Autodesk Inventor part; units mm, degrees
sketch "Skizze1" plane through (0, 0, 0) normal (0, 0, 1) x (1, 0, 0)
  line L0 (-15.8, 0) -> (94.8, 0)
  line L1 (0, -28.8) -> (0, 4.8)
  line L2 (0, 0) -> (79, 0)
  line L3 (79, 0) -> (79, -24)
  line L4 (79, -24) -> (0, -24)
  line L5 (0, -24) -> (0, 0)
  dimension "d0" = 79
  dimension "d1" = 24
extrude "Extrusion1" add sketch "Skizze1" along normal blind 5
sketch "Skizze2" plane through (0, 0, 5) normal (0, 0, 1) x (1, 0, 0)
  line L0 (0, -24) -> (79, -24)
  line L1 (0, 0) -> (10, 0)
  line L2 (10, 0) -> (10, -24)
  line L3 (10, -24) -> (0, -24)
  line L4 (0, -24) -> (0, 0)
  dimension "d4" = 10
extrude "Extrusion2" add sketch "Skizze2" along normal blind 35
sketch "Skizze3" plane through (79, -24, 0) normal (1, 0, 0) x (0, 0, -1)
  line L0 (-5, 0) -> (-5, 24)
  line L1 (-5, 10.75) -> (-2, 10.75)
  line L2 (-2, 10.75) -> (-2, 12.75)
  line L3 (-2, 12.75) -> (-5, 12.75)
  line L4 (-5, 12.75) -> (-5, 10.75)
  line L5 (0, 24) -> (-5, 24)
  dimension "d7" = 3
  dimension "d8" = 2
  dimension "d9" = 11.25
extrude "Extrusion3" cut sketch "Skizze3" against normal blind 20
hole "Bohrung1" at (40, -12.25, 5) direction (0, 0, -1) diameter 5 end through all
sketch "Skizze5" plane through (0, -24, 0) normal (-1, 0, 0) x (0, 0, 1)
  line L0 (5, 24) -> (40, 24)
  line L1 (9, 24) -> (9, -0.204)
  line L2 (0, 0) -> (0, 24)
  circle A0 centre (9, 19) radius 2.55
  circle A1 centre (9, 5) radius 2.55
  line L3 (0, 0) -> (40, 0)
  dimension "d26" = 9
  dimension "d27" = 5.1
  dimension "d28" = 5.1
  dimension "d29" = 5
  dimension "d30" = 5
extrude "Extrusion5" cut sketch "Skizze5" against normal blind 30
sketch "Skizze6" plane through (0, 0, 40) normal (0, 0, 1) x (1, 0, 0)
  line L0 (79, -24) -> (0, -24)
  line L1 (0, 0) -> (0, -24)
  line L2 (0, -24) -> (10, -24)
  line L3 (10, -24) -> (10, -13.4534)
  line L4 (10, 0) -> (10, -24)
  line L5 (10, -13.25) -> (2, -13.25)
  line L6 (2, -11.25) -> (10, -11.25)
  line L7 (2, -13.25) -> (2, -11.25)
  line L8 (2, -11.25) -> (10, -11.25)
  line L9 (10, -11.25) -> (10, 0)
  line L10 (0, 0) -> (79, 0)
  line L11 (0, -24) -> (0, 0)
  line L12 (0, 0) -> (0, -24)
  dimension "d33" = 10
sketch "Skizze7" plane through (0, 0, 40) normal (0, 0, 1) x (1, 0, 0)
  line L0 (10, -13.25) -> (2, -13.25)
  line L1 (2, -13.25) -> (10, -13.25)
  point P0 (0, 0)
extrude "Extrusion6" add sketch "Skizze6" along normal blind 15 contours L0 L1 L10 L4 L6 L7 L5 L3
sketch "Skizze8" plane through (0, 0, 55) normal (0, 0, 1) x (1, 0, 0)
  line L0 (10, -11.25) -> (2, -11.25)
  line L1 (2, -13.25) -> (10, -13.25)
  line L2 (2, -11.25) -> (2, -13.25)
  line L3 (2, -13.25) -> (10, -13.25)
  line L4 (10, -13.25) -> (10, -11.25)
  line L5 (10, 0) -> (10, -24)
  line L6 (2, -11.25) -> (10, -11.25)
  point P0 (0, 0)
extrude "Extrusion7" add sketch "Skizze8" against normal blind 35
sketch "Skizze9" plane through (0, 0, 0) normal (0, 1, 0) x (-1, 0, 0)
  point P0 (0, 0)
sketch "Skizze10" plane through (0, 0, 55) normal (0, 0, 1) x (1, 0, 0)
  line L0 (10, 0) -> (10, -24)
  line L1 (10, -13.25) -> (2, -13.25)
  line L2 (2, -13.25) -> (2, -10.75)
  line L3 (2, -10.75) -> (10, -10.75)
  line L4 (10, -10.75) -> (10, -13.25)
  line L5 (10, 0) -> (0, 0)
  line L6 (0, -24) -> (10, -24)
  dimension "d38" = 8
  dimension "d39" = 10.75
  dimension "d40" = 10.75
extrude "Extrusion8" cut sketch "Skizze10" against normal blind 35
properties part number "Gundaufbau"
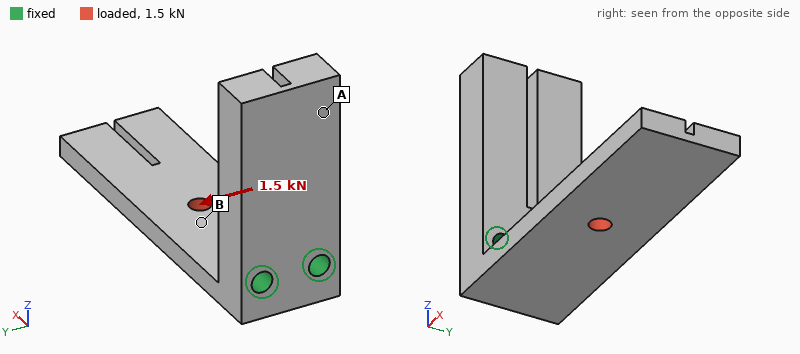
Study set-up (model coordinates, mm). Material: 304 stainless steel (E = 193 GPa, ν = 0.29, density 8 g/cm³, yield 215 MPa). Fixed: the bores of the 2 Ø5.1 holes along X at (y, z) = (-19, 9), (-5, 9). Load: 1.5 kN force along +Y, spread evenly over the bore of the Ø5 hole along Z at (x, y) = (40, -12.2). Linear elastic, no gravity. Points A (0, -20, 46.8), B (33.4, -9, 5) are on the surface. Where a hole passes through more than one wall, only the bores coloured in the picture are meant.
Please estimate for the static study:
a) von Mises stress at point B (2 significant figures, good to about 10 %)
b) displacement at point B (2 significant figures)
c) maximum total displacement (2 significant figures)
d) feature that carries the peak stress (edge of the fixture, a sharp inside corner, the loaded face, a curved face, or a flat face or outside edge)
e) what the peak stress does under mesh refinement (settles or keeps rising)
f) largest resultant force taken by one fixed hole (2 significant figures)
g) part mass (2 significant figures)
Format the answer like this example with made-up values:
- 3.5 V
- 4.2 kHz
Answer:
- 30 MPa
- 25 µm
- 73 µm
- edge of the fixture
- keeps rising
- 2.8 kN
- 160 g
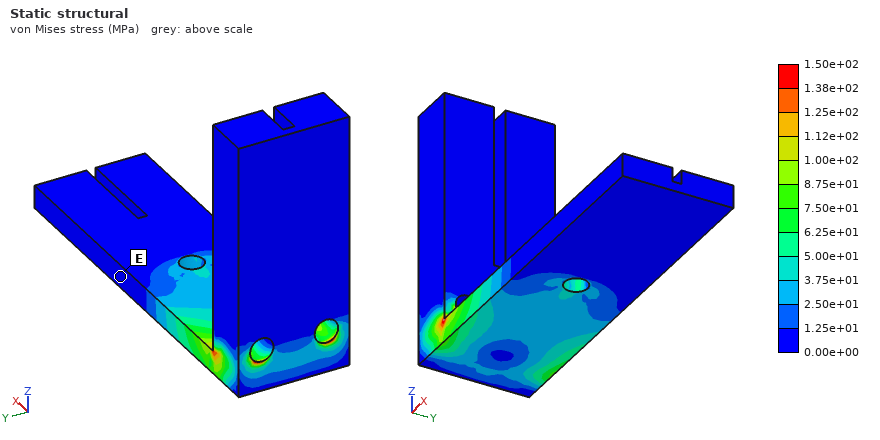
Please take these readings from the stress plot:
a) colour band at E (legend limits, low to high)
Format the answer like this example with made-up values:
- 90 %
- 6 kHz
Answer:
- 0.00e+00 to 1.25e+01 MPa
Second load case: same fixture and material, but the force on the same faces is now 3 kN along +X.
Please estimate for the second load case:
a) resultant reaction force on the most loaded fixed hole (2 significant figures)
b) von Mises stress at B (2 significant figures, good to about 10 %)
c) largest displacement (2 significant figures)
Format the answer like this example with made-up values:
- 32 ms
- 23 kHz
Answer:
- 1.5 kN
- 33 MPa
- 21 µm
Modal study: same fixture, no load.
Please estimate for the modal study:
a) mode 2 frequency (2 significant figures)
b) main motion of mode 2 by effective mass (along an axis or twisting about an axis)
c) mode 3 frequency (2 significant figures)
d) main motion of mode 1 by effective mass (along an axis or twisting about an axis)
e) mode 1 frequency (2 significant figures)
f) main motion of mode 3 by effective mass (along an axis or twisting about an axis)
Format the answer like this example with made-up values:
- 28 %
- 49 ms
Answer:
- 3000 Hz
- along Y
- 3900 Hz
- along Z
- 780 Hz
- along X
